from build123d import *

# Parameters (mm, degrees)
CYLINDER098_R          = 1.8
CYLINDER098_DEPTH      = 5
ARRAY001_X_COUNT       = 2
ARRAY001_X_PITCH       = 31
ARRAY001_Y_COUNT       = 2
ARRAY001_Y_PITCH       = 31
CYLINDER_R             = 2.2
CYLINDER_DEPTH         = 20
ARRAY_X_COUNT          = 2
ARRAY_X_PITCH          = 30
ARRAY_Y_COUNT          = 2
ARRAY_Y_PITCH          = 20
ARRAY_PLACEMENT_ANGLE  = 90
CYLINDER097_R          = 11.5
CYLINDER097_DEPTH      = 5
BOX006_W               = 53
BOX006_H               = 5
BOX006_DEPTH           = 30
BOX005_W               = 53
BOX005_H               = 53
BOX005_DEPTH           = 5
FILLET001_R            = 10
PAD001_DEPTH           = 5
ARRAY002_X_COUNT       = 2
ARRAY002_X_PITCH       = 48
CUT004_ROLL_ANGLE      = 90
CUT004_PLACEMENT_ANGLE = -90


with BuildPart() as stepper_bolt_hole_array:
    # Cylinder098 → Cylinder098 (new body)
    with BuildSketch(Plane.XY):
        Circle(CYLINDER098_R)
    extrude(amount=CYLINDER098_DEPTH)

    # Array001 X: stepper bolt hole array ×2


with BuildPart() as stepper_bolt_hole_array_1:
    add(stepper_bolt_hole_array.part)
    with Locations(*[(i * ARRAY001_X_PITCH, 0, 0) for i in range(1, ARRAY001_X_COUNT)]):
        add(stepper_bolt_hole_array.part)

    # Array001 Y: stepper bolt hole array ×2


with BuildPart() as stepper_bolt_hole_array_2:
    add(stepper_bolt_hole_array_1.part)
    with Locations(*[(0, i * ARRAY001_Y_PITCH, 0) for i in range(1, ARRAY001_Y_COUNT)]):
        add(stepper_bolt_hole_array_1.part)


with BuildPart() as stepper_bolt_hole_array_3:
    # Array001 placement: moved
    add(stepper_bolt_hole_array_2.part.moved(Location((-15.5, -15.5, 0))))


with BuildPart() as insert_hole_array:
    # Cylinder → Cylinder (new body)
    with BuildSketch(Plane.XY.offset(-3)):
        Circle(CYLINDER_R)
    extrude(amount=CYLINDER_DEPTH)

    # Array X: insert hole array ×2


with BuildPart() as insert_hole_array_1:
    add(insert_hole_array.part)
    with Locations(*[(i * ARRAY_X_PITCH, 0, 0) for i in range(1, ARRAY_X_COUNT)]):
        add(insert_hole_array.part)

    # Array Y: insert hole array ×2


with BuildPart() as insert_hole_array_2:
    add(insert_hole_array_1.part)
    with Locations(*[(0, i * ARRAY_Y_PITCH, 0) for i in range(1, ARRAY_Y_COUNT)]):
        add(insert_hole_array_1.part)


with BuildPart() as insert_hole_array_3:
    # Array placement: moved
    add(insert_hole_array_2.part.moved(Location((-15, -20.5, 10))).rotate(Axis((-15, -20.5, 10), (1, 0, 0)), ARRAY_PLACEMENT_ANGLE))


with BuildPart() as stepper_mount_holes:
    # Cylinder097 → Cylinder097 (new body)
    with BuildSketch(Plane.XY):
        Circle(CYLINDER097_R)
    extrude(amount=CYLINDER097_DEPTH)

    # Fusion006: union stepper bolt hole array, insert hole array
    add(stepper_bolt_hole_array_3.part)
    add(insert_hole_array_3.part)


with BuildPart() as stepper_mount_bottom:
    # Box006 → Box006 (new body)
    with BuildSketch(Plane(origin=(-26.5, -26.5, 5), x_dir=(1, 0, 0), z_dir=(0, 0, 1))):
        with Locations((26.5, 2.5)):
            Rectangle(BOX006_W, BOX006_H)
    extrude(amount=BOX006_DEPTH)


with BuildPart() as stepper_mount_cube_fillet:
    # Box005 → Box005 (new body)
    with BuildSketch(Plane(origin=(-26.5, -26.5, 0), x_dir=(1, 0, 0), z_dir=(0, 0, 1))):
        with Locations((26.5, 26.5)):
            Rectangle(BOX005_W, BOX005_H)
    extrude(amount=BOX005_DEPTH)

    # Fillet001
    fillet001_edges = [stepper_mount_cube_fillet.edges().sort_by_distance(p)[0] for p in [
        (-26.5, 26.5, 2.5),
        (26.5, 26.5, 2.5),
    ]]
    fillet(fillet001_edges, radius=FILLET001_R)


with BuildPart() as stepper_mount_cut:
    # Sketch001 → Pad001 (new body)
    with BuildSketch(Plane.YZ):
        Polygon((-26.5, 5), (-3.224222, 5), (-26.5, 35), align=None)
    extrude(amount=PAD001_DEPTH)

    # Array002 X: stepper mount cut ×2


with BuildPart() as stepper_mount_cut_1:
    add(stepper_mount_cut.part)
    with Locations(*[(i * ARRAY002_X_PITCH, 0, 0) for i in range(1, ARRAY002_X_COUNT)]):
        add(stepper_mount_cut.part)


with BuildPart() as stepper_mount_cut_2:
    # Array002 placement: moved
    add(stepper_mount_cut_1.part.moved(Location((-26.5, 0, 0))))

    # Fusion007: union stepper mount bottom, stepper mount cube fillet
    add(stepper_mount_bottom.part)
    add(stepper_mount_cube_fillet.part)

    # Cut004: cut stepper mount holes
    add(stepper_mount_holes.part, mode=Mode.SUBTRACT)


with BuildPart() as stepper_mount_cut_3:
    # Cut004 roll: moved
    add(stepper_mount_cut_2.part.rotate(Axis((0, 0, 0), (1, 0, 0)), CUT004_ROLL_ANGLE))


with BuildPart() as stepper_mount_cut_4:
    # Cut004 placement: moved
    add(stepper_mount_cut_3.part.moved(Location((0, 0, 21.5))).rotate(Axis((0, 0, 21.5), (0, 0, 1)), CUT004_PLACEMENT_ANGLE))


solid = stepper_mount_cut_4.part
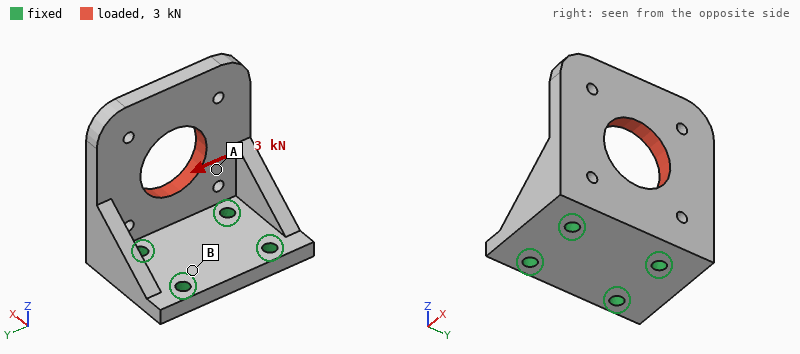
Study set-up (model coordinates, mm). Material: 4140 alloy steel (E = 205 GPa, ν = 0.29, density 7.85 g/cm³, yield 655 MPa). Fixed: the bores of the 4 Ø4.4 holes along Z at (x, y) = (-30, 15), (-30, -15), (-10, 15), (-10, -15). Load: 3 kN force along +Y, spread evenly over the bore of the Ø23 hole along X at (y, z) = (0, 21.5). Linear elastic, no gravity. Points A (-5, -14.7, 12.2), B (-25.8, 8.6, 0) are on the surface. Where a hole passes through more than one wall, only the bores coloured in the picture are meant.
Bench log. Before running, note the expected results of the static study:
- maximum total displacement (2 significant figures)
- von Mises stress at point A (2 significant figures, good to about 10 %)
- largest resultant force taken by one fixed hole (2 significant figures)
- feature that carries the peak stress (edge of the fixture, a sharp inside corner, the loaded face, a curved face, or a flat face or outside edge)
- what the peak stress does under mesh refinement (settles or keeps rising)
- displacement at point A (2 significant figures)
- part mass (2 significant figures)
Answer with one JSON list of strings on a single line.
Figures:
["36 µm", "31 MPa", "2.7 kN", "edge of the fixture", "keeps rising", "12 µm", "170 g"]
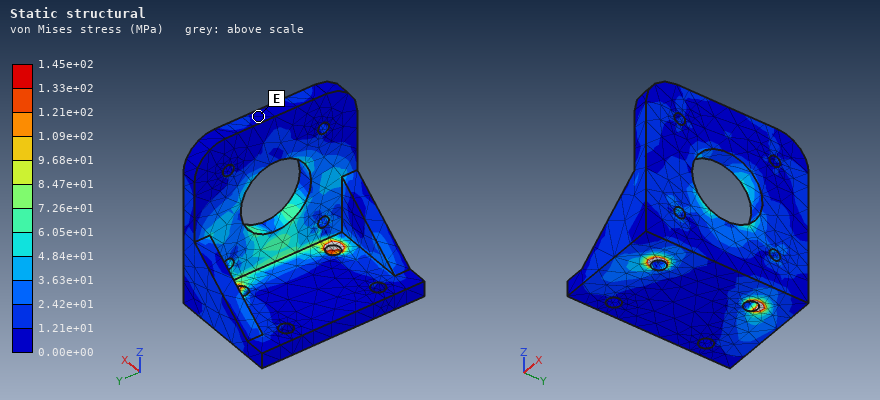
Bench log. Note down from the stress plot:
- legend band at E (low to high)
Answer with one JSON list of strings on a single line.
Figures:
["0.00e+00 to 1.21e+01 MPa"]
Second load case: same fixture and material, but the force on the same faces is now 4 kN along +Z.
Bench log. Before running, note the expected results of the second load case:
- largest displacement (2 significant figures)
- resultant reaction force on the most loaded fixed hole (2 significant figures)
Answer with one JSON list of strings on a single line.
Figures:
["28 µm", "2.4 kN"]
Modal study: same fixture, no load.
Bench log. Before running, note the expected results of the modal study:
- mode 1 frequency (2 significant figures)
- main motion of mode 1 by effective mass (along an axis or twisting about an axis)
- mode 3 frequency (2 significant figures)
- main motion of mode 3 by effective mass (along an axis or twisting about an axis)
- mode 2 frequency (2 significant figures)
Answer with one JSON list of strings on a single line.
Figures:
["2200 Hz", "along X", "6400 Hz", "along Y", "4600 Hz"]
